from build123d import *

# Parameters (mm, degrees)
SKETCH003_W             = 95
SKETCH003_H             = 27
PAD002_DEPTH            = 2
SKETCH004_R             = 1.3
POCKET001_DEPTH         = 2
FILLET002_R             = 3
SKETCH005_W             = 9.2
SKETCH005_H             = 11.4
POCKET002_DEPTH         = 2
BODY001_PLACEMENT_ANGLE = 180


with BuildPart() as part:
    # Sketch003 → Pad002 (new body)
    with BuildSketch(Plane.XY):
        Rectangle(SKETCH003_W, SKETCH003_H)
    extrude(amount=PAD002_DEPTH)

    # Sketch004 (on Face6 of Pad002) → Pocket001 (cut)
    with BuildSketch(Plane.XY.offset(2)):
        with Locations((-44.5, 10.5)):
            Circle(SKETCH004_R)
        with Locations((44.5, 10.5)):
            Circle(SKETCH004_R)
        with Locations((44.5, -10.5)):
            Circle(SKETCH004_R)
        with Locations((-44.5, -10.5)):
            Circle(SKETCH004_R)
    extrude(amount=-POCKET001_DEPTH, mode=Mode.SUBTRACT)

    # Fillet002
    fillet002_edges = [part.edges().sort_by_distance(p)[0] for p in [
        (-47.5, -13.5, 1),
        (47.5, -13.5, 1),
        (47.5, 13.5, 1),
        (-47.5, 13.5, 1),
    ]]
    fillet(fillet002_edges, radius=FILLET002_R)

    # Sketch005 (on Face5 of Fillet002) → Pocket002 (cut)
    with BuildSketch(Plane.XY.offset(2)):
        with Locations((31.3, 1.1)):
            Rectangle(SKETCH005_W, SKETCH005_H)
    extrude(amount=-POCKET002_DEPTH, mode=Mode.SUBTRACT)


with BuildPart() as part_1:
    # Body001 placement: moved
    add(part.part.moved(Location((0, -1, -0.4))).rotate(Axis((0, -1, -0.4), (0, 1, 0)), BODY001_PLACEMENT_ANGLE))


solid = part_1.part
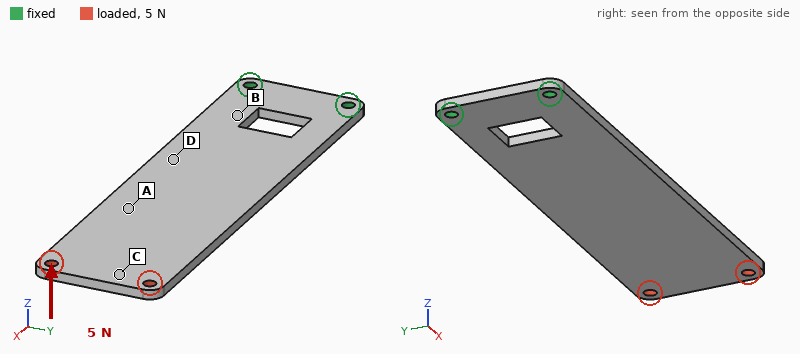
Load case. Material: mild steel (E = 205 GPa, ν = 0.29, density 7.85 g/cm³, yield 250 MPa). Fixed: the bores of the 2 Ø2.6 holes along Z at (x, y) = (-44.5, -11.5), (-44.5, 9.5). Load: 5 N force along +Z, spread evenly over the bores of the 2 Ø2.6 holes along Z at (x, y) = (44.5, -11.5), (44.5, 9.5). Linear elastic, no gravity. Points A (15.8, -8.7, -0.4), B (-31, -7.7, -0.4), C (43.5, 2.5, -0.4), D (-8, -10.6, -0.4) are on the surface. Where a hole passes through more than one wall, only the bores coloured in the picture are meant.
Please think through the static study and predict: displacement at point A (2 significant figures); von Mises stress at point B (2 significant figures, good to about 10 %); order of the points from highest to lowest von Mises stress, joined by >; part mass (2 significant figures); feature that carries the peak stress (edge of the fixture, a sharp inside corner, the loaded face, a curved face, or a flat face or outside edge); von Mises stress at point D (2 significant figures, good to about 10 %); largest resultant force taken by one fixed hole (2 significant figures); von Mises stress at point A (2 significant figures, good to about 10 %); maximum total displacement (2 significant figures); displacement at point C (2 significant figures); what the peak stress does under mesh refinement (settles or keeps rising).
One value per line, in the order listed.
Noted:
0.23 mm
36 MPa
B > D > A > C
38 g
edge of the fixture
15 MPa
2.6 N
8.0 MPa
0.43 mm
0.40 mm
keeps rising
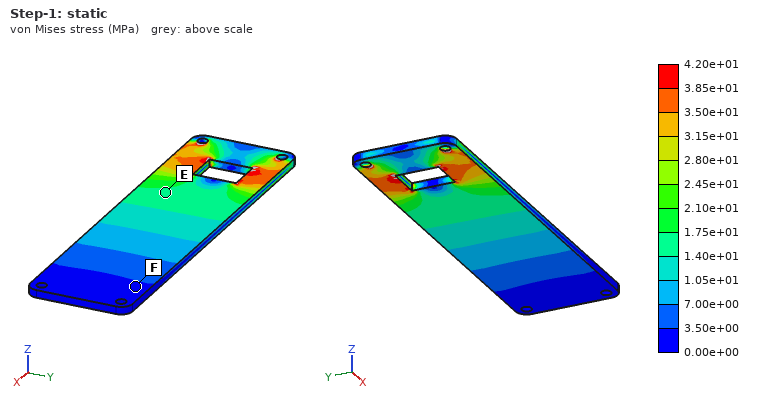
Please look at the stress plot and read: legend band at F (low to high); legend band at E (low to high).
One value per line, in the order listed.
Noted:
0.00e+00 to 3.50e+00 MPa
1.40e+01 to 1.75e+01 MPa
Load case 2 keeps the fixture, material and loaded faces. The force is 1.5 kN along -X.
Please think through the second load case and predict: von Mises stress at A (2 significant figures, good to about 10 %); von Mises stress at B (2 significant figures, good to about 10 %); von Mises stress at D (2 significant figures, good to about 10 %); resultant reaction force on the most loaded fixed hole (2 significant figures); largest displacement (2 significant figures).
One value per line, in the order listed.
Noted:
28 MPa
50 MPa
29 MPa
760 N
18 µm
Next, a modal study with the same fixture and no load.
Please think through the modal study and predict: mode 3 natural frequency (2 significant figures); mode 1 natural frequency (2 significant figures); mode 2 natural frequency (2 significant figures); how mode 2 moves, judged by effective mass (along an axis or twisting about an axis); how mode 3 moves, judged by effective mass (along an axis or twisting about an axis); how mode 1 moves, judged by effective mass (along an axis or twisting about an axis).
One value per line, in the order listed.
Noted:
1300 Hz
170 Hz
1200 Hz
along Z
twisting about X
along Z
